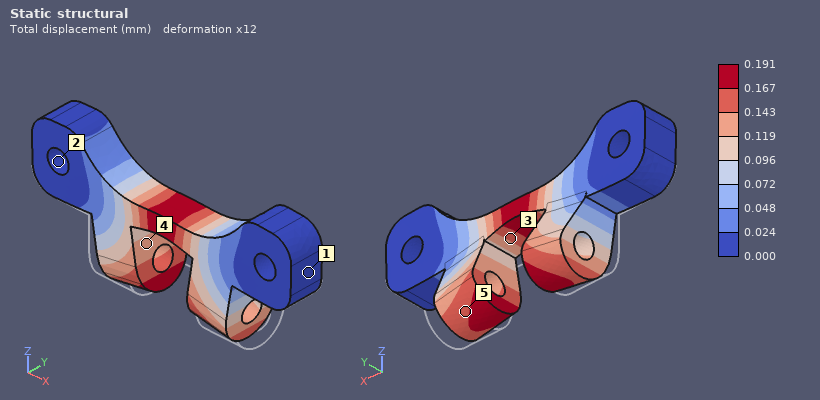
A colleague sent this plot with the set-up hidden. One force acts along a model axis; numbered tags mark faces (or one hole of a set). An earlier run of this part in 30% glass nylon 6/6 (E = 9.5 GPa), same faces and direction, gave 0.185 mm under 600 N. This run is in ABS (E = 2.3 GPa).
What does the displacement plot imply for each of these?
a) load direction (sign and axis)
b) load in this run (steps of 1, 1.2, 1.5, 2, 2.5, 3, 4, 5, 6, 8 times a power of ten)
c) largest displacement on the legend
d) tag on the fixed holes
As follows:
+Z
150 N
0.191 mm
2
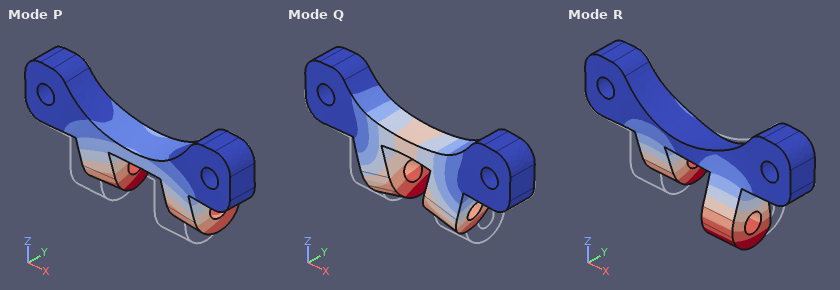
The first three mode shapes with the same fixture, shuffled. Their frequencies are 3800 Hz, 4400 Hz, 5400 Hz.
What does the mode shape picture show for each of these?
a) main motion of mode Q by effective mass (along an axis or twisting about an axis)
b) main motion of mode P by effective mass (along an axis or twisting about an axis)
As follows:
along Z
along Y
